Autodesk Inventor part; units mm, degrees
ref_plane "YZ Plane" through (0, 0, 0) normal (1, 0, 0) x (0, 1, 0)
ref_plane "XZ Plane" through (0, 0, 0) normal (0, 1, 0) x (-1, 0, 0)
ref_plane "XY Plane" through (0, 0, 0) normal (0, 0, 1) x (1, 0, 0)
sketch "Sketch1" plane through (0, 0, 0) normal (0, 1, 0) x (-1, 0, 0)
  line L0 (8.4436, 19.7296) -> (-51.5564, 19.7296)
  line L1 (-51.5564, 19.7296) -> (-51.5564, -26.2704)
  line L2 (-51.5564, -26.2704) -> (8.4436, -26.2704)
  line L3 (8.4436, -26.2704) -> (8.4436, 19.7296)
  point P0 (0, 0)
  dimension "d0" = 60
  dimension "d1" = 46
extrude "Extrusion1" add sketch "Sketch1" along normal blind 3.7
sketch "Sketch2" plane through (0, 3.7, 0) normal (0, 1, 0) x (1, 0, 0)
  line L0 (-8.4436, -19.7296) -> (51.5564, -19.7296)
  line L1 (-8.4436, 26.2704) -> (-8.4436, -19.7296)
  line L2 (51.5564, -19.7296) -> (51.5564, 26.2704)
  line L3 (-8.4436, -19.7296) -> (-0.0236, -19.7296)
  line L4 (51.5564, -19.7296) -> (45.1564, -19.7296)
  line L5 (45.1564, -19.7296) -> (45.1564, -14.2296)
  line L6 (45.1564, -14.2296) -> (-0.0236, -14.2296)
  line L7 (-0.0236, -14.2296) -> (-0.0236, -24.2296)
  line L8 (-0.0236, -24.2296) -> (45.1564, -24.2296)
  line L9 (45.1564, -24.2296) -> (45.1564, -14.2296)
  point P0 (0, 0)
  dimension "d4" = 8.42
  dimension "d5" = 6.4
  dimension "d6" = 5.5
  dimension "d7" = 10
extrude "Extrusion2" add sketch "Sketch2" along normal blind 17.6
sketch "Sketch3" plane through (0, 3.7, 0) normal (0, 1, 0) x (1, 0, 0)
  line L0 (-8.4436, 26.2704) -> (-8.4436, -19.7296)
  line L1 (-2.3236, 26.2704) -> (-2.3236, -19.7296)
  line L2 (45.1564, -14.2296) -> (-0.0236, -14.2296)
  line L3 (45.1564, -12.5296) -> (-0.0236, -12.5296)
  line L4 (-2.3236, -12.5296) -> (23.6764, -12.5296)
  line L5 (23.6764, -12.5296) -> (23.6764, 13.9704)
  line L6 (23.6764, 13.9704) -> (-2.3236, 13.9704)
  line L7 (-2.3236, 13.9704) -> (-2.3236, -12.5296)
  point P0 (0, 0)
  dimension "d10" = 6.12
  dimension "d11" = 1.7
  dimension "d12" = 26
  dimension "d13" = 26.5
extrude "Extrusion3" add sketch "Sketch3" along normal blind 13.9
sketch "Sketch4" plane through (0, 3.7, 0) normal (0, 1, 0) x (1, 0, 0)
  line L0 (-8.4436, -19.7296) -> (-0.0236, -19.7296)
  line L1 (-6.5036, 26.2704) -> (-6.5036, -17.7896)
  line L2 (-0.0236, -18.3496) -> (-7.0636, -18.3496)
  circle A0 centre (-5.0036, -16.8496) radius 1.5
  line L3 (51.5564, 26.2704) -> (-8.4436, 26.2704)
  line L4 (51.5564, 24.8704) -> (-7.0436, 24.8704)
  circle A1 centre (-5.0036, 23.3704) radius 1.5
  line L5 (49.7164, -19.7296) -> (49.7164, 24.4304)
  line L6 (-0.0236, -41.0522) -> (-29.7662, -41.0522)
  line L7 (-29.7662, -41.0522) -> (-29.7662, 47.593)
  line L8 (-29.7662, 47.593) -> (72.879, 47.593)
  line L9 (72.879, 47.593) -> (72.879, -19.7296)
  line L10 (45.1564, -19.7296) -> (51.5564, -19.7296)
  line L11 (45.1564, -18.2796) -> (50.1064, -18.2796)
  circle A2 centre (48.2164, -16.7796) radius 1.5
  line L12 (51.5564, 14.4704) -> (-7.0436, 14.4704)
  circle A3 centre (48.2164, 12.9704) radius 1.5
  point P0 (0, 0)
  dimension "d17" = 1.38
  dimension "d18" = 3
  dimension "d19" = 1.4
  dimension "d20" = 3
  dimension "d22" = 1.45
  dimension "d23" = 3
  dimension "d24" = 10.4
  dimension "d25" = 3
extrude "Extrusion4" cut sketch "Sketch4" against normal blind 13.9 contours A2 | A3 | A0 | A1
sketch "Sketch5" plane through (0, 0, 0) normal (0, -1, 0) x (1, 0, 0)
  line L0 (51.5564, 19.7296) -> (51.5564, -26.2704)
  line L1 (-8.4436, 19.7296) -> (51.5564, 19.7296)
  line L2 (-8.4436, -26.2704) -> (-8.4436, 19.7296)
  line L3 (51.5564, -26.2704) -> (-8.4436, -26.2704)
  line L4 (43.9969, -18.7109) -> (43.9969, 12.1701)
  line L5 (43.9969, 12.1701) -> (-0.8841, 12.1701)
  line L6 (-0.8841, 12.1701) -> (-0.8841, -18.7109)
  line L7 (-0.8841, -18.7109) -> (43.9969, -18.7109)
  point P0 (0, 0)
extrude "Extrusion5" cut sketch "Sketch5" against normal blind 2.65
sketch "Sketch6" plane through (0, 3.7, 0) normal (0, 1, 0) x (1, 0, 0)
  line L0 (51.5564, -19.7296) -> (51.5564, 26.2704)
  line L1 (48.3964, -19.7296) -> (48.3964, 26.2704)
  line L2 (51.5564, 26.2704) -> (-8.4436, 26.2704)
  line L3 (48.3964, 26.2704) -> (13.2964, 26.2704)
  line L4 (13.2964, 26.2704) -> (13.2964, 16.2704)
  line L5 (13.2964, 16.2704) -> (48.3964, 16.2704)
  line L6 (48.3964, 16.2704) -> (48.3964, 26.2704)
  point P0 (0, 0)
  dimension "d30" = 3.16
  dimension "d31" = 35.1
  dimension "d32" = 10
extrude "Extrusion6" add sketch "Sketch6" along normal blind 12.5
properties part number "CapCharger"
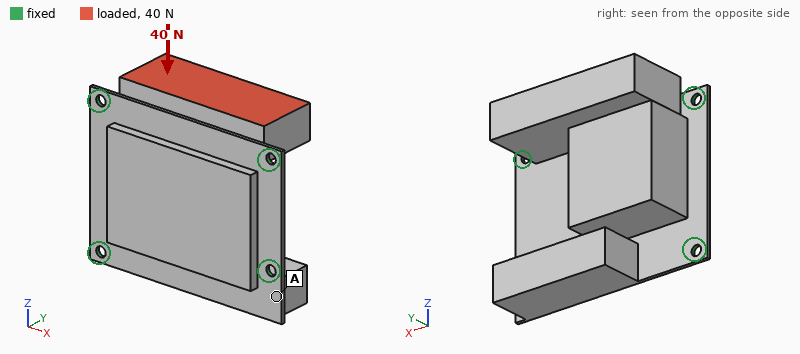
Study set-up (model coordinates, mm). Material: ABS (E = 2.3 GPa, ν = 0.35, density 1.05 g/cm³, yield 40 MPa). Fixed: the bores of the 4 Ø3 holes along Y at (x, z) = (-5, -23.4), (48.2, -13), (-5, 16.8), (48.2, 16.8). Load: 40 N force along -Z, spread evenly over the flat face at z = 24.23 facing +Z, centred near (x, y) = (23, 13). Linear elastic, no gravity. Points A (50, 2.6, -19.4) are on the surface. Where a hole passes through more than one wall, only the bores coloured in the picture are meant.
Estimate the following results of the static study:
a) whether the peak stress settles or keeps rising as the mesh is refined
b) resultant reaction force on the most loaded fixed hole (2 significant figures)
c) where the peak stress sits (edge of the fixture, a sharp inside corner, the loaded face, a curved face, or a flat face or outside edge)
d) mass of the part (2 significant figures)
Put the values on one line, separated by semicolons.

keeps rising; 17 N; edge of the fixture; 30 g
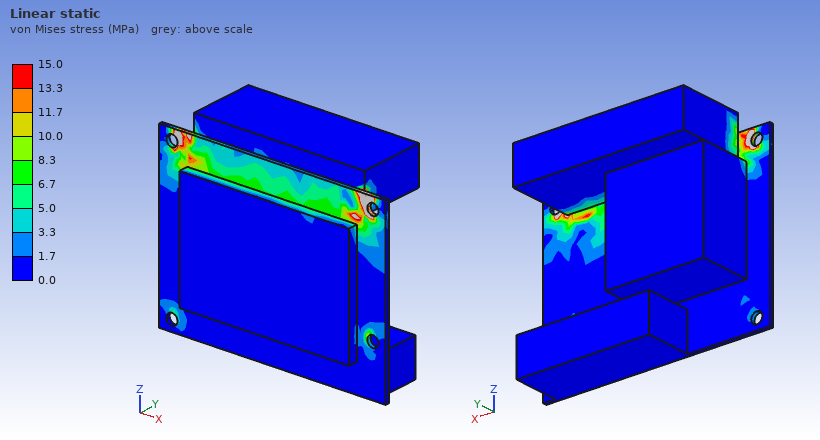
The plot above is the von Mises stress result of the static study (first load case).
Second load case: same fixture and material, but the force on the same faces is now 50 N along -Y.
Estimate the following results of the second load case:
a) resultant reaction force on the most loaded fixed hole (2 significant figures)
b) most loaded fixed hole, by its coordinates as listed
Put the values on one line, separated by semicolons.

40 N; (48.2, 16.8)
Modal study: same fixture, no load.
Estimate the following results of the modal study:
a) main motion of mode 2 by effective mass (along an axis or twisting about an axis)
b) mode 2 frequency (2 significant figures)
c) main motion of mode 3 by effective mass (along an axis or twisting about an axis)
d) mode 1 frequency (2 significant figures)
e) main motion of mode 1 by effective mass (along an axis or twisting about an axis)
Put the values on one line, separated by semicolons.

along Y; 680 Hz; along Y; 480 Hz; along Z
